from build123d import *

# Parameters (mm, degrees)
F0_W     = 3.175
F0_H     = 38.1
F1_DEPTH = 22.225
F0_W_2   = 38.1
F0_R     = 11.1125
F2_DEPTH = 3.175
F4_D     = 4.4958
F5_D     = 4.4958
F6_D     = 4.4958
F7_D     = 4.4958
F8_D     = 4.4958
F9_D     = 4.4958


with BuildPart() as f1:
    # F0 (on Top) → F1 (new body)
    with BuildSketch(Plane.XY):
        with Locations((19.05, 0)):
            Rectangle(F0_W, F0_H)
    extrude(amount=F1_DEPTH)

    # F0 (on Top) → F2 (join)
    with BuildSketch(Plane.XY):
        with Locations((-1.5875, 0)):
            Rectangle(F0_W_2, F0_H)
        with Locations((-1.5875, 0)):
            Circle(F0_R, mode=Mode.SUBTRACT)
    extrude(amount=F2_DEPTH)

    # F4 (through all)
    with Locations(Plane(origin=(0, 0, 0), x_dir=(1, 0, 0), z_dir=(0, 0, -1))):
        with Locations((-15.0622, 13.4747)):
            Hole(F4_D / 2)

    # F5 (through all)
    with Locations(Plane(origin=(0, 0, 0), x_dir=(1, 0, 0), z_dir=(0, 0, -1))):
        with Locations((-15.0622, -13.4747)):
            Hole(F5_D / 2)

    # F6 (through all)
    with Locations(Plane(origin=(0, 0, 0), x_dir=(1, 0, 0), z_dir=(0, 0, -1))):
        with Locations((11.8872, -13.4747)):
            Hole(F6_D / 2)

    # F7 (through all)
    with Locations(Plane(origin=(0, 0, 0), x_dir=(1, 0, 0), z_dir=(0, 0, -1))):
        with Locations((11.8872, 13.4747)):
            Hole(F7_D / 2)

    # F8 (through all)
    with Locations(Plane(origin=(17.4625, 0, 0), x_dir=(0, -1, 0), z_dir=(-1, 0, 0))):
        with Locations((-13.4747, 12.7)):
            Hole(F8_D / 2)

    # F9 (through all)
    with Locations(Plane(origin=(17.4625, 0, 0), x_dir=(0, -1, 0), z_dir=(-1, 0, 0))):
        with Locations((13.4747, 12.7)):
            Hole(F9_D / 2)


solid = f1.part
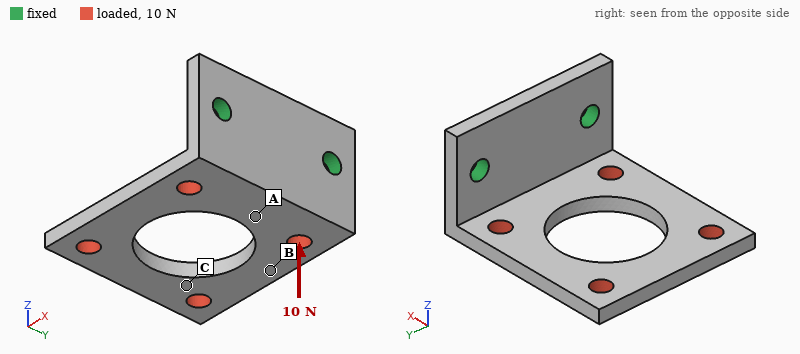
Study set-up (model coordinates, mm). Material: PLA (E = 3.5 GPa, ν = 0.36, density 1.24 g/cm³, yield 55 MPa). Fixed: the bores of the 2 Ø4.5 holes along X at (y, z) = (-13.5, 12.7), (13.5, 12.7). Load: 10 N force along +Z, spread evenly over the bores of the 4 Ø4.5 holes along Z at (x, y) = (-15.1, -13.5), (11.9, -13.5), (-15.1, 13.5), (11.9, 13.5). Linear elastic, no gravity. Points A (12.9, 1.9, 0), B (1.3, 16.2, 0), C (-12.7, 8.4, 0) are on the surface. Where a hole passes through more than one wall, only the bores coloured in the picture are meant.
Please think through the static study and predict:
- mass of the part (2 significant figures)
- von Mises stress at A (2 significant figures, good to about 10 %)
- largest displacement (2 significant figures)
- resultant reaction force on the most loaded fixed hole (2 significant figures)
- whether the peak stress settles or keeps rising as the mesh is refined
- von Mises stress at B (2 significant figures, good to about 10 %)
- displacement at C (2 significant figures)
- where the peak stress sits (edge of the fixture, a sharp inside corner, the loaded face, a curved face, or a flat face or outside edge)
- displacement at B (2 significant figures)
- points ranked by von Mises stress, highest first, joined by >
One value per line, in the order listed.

7.1 g
1.7 MPa
0.61 mm
5.1 N
keeps rising
2.9 MPa
0.45 mm
edge of the fixture
0.20 mm
B > A > C
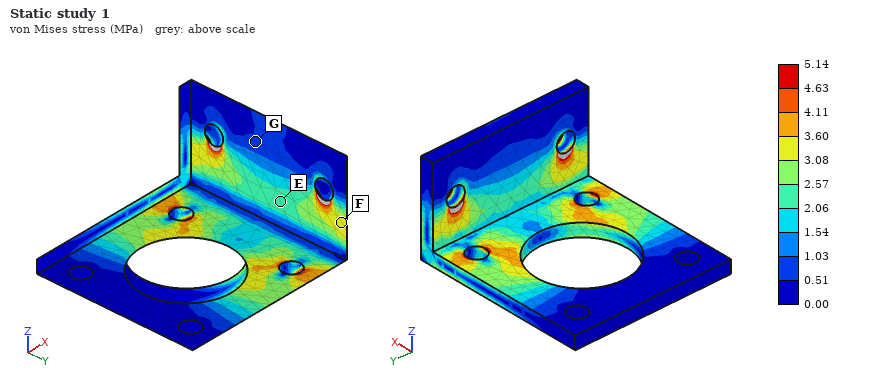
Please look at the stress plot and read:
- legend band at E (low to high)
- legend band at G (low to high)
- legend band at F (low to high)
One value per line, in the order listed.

2.06 to 2.57 MPa
0.51 to 1.03 MPa
3.08 to 3.60 MPa
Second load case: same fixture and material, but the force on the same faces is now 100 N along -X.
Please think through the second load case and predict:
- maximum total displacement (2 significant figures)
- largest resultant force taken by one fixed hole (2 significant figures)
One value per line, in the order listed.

0.63 mm
50 N
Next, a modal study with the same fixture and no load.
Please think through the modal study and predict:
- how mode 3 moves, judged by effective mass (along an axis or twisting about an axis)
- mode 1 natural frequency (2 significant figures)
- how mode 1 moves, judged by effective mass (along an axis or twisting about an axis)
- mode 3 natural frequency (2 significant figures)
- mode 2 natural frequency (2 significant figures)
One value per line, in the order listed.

along Y
390 Hz
along Z
1400 Hz
980 Hz
